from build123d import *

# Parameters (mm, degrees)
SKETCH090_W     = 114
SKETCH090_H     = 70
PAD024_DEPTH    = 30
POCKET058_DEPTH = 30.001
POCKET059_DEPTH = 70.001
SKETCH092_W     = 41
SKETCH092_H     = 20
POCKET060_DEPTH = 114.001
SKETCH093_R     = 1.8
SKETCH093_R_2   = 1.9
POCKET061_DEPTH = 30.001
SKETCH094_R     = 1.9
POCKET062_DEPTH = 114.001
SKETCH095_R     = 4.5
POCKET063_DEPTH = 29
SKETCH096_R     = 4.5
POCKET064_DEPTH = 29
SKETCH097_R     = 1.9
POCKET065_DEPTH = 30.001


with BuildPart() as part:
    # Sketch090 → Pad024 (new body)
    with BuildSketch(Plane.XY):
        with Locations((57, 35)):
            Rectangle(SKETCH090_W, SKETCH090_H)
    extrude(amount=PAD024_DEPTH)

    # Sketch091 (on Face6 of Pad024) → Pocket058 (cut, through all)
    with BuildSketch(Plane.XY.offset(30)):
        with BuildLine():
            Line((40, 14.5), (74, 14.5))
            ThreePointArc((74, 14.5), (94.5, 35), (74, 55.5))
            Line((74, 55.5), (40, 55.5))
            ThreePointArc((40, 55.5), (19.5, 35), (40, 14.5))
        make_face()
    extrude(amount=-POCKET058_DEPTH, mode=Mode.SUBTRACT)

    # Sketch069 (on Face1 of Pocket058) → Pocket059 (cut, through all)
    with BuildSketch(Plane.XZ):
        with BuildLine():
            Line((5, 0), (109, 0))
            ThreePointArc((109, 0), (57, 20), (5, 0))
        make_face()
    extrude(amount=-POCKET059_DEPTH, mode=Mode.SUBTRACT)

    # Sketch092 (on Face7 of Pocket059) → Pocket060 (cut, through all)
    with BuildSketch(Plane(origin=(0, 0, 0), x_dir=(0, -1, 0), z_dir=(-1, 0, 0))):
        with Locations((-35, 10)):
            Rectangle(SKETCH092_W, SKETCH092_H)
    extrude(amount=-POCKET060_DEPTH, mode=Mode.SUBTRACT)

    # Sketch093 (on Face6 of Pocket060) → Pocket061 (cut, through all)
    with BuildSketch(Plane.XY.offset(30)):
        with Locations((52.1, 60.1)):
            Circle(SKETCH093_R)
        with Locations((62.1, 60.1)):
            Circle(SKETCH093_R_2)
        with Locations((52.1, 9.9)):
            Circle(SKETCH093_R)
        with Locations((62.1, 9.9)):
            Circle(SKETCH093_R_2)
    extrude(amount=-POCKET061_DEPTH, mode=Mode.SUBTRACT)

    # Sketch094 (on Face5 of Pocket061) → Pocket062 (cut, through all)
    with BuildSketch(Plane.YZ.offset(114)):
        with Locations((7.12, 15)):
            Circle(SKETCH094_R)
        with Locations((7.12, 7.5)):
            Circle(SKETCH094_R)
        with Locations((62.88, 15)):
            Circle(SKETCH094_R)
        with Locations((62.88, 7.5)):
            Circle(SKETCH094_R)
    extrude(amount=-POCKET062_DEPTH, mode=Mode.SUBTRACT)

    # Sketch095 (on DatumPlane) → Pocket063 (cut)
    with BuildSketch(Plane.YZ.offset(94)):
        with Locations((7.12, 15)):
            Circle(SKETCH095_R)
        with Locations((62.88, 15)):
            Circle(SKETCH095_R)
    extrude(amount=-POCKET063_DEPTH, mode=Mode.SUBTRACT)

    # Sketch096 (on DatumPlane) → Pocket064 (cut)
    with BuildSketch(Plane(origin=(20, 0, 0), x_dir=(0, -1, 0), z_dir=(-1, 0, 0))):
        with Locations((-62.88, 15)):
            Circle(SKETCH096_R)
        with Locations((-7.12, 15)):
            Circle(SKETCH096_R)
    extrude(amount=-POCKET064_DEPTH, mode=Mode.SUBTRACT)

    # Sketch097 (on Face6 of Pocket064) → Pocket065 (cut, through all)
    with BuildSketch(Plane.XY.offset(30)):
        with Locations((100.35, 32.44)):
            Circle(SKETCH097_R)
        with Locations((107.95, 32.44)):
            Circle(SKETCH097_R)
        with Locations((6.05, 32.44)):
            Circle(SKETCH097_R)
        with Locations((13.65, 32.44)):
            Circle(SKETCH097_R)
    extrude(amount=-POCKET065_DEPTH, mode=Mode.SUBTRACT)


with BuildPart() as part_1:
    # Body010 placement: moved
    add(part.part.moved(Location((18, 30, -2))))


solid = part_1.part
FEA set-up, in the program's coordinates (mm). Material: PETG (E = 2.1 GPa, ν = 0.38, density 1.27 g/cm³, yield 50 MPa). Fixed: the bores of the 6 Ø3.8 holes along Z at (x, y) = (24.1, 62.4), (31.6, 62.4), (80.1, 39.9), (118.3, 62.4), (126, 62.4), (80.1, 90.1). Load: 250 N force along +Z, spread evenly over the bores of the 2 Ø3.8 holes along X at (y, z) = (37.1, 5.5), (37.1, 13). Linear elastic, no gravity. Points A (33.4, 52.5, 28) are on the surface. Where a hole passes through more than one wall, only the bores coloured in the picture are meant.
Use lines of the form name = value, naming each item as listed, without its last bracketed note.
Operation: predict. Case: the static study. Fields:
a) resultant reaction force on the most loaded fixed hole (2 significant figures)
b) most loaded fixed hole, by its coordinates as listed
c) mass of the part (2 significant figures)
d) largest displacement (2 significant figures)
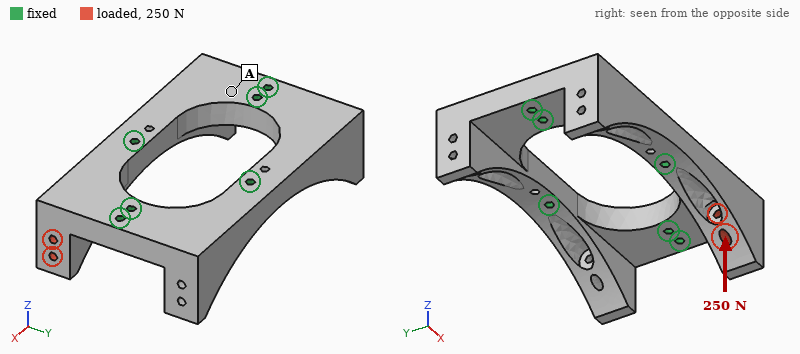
resultant reaction force on the most loaded fixed hole = 160 N
most loaded fixed hole, by its coordinates as listed = (126, 62.4)
mass of the part = 92 g
largest displacement = 0.49 mm
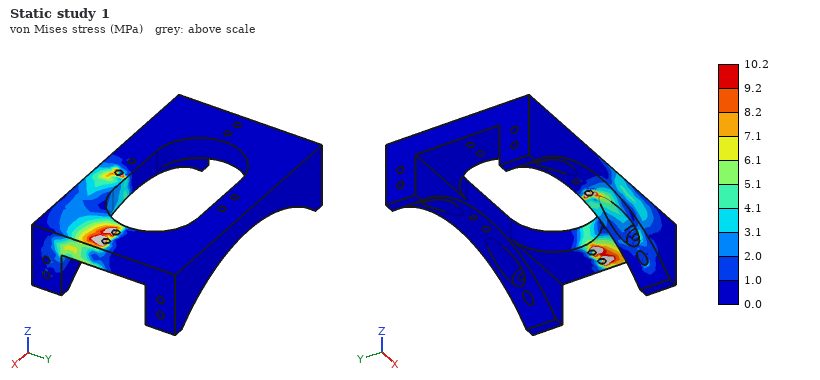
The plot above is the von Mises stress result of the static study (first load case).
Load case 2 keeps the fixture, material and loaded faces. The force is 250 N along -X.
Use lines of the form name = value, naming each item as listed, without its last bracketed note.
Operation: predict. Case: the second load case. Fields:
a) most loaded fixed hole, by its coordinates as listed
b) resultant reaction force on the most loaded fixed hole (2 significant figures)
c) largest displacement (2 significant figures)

most loaded fixed hole, by its coordinates as listed = (80.1, 39.9)
resultant reaction force on the most loaded fixed hole = 200 N
largest displacement = 0.20 mm
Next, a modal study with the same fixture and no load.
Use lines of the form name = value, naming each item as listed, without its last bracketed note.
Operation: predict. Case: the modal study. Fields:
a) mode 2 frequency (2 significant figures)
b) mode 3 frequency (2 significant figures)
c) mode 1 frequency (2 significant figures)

mode 2 frequency = 1100 Hz
mode 3 frequency = 1200 Hz
mode 1 frequency = 1000 Hz
